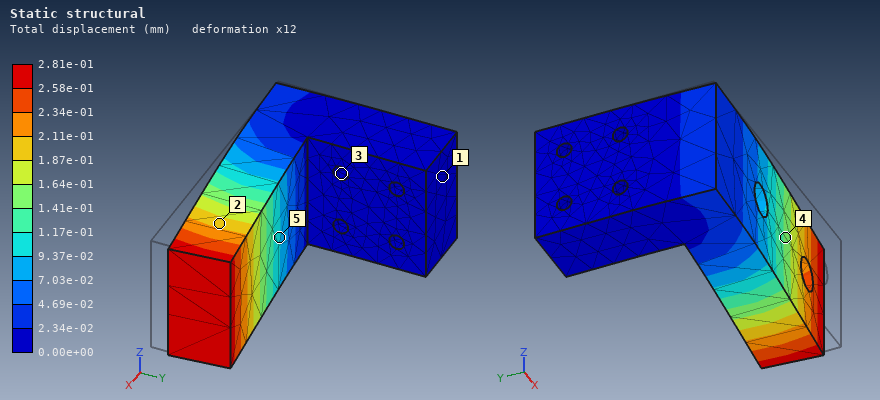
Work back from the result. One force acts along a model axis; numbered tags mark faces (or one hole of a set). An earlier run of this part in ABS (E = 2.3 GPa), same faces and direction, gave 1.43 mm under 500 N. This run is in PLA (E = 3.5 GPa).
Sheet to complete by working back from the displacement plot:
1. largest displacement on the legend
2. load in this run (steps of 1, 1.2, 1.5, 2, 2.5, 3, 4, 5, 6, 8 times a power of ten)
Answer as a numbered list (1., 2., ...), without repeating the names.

1. 2.81e-01 mm
2. 150 N
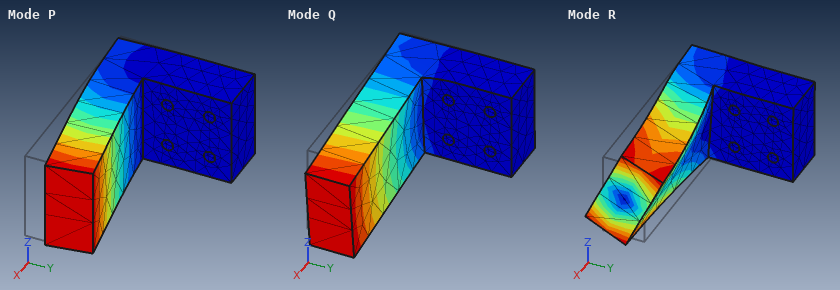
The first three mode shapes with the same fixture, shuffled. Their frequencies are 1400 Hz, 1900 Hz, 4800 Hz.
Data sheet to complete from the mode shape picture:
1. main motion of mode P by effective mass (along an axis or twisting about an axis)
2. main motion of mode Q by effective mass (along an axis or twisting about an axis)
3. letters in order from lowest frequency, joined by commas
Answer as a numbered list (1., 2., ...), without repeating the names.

1. along Y
2. along Z
3. P, Q, R
